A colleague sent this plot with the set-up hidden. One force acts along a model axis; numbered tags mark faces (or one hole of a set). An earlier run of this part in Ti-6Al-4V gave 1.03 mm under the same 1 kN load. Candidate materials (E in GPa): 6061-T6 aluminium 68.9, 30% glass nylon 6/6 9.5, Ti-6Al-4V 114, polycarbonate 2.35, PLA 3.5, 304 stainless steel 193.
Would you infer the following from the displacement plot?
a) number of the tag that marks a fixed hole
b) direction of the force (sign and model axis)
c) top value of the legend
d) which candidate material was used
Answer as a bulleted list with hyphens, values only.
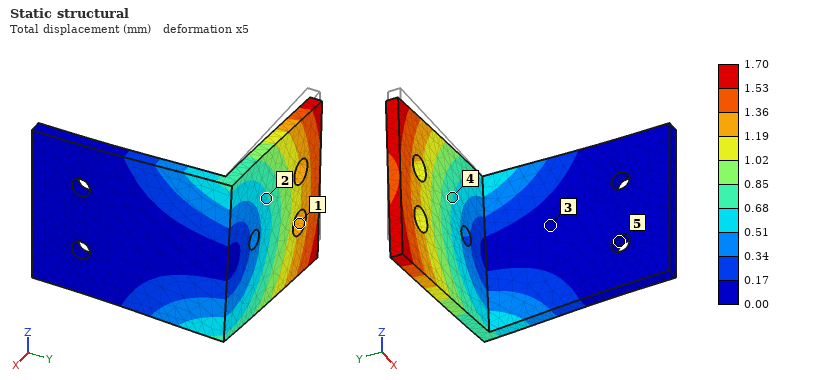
- 5
- -Z
- 1.70 mm
- 6061-T6 aluminium
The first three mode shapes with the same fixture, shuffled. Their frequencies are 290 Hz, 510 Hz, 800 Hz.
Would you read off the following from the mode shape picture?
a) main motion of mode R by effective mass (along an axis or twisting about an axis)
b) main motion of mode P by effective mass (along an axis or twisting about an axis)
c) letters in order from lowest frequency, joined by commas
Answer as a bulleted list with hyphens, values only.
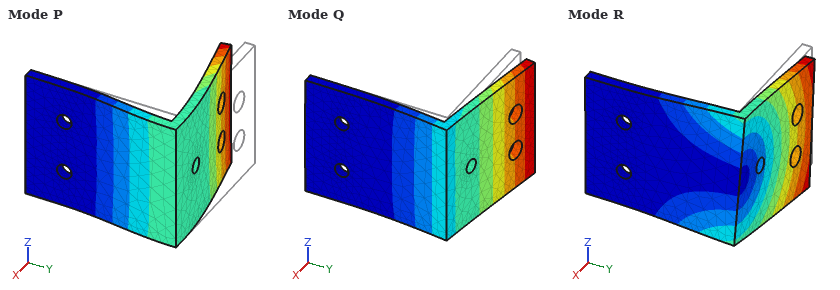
- along Z
- along X
- Q, R, P
